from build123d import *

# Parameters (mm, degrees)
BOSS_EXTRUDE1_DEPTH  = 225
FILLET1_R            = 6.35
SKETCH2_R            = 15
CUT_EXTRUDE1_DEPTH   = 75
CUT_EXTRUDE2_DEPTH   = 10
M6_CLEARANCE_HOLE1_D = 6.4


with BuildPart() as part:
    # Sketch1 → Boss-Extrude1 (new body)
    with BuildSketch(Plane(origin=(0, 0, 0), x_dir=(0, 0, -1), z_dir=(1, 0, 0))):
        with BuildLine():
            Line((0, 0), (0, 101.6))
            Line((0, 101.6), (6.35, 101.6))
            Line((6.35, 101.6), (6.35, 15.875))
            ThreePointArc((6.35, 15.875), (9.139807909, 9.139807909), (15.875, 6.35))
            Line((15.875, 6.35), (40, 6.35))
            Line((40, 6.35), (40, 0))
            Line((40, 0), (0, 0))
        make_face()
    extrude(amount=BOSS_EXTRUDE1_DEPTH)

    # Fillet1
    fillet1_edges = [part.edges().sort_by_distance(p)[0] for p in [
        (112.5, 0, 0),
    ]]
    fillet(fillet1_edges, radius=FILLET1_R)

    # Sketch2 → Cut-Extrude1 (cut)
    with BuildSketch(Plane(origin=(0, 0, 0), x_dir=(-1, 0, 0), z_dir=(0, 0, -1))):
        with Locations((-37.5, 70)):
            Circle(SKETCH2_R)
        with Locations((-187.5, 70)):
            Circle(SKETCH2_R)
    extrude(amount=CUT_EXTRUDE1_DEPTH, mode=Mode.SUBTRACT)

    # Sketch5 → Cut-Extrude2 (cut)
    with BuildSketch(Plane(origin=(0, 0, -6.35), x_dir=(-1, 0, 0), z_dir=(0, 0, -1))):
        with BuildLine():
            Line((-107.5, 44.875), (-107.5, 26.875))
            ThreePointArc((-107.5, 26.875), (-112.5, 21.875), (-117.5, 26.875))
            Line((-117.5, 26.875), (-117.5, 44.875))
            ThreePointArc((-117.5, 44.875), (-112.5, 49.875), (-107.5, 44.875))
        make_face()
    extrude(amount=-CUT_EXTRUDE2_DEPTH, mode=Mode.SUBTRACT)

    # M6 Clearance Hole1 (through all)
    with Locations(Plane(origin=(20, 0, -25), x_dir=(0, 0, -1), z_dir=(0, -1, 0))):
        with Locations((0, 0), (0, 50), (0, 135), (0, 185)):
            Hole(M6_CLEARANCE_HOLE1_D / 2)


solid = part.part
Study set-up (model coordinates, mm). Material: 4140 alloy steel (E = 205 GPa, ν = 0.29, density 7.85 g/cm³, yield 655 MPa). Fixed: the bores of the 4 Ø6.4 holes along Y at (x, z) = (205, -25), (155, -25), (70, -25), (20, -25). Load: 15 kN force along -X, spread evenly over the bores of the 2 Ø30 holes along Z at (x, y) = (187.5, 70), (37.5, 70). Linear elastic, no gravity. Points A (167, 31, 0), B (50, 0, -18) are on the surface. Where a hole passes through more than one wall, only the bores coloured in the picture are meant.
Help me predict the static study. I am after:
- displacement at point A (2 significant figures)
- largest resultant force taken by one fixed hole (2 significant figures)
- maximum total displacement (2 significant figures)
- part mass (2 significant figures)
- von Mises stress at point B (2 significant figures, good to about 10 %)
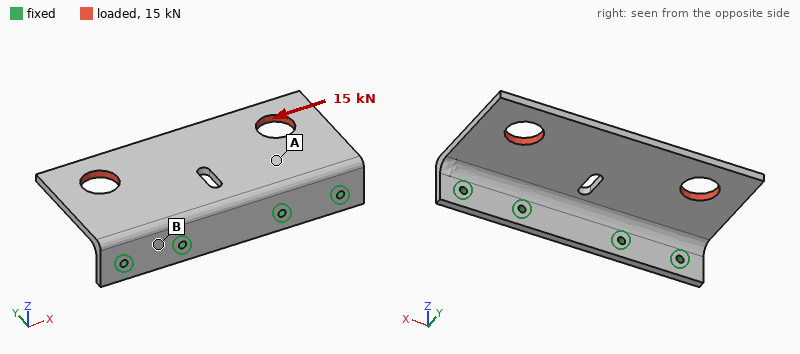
0.073 mm
5.7 kN
0.28 mm
1.4 kg
47 MPa
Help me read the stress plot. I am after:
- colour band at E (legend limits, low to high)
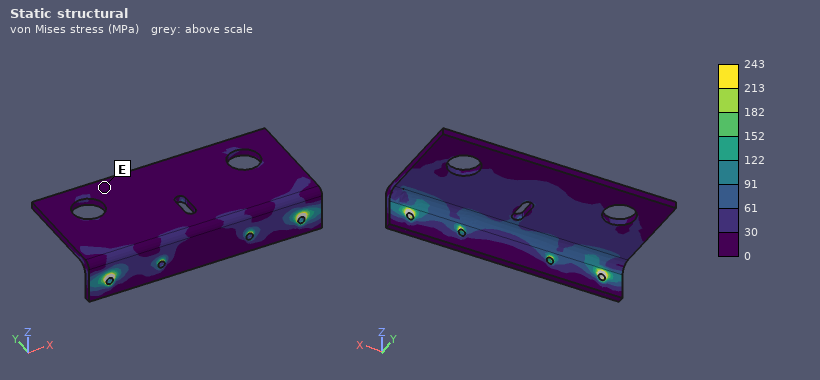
0 to 30 MPa
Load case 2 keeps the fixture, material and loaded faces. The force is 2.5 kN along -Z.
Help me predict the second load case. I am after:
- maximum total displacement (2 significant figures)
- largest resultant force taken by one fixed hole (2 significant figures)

0.70 mm
720 N
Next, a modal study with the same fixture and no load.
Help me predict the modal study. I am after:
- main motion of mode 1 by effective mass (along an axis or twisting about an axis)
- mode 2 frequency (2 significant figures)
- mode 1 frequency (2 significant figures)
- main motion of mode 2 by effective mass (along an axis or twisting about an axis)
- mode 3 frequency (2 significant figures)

along Z
720 Hz
450 Hz
twisting about Y
1400 Hz
